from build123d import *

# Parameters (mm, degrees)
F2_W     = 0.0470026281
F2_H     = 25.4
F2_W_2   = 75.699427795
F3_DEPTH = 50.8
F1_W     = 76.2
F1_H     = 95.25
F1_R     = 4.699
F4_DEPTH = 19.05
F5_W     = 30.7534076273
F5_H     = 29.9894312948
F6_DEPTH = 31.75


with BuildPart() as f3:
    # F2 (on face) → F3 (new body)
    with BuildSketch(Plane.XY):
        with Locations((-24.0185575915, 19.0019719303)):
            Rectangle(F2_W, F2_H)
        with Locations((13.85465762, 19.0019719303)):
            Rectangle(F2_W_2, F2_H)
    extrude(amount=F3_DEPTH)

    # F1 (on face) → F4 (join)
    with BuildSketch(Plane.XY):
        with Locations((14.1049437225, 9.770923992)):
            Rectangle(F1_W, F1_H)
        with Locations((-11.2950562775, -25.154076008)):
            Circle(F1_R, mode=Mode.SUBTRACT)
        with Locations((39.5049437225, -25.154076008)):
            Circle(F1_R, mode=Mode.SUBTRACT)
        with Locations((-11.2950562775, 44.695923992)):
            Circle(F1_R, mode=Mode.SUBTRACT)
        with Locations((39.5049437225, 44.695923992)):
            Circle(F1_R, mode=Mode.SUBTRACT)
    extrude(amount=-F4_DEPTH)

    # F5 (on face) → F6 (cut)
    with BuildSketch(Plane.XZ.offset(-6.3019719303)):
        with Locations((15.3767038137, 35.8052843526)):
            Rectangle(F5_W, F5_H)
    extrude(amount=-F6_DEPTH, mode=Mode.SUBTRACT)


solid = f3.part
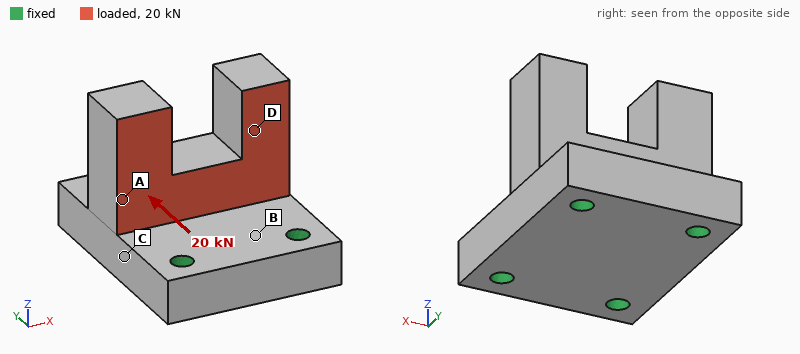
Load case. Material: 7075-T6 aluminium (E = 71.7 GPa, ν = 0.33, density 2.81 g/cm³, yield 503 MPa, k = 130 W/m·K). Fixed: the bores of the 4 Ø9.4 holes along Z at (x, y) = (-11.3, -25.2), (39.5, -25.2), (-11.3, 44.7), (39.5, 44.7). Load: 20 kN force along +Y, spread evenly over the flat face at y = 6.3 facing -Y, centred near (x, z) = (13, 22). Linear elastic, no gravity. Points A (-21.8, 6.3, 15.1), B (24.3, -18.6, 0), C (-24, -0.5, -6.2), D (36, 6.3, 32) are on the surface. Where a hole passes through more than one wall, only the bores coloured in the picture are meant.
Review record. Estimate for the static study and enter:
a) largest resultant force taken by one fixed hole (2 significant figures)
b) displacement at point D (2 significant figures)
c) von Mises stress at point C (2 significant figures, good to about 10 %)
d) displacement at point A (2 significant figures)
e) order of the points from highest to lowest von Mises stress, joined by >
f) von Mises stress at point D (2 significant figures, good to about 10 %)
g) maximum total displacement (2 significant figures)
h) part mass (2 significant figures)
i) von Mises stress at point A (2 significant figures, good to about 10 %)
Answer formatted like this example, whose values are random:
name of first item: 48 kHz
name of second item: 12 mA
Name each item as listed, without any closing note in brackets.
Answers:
largest resultant force taken by one fixed hole: 8.2 kN
displacement at point D: 0.077 mm
von Mises stress at point C: 27 MPa
displacement at point A: 0.046 mm
order of the points from highest to lowest von Mises stress, joined by >: A > C > D > B
von Mises stress at point D: 16 MPa
maximum total displacement: 0.12 mm
part mass: 580 g
von Mises stress at point A: 34 MPa
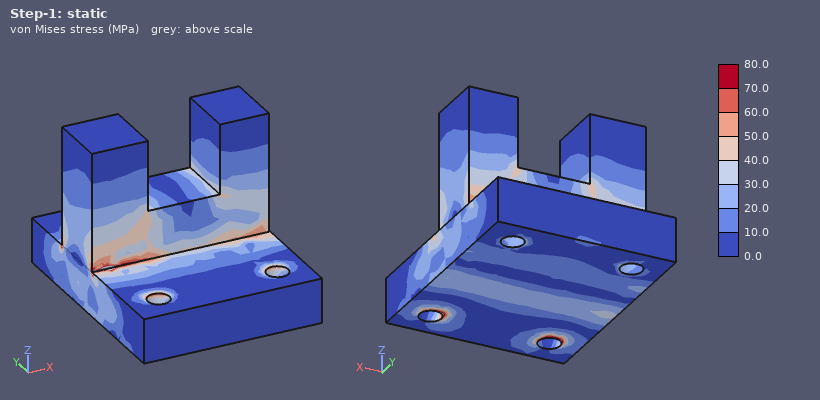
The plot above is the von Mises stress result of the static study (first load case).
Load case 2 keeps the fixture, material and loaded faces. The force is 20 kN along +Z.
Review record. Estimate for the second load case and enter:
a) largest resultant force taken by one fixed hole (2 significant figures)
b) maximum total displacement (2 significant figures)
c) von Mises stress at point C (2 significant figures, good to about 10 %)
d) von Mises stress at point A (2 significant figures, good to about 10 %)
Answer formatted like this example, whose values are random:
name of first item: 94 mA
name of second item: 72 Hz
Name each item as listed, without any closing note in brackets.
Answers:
largest resultant force taken by one fixed hole: 5.8 kN
maximum total displacement: 86 µm
von Mises stress at point C: 29 MPa
von Mises stress at point A: 35 MPa
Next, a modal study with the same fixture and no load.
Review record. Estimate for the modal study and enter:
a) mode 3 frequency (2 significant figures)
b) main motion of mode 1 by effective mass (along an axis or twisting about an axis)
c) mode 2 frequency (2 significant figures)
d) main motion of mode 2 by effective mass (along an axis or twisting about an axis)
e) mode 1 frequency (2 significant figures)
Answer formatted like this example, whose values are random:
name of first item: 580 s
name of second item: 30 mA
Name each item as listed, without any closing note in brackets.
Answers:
mode 3 frequency: 6700 Hz
main motion of mode 1 by effective mass: along Y
mode 2 frequency: 5900 Hz
main motion of mode 2 by effective mass: along X
mode 1 frequency: 5600 Hz
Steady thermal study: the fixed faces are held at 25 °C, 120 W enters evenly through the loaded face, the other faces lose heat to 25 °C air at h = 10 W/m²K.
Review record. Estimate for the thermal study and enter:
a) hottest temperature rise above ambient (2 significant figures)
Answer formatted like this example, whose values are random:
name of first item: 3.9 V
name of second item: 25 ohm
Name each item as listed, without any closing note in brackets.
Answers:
hottest temperature rise above ambient: 27 K
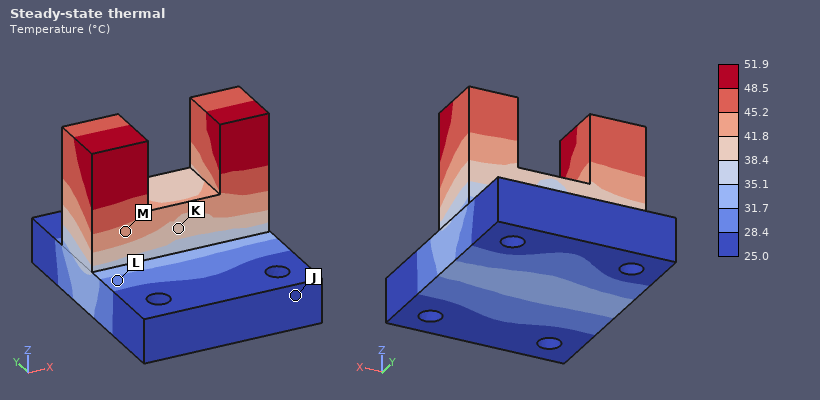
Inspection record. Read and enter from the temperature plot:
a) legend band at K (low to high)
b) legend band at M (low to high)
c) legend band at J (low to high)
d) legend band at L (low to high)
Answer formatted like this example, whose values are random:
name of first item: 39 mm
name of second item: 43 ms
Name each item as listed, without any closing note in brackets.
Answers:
legend band at K: 38.4 to 41.8 °C
legend band at M: 41.8 to 45.2 °C
legend band at J: 25.0 to 28.4 °C
legend band at L: 28.4 to 31.7 °C
